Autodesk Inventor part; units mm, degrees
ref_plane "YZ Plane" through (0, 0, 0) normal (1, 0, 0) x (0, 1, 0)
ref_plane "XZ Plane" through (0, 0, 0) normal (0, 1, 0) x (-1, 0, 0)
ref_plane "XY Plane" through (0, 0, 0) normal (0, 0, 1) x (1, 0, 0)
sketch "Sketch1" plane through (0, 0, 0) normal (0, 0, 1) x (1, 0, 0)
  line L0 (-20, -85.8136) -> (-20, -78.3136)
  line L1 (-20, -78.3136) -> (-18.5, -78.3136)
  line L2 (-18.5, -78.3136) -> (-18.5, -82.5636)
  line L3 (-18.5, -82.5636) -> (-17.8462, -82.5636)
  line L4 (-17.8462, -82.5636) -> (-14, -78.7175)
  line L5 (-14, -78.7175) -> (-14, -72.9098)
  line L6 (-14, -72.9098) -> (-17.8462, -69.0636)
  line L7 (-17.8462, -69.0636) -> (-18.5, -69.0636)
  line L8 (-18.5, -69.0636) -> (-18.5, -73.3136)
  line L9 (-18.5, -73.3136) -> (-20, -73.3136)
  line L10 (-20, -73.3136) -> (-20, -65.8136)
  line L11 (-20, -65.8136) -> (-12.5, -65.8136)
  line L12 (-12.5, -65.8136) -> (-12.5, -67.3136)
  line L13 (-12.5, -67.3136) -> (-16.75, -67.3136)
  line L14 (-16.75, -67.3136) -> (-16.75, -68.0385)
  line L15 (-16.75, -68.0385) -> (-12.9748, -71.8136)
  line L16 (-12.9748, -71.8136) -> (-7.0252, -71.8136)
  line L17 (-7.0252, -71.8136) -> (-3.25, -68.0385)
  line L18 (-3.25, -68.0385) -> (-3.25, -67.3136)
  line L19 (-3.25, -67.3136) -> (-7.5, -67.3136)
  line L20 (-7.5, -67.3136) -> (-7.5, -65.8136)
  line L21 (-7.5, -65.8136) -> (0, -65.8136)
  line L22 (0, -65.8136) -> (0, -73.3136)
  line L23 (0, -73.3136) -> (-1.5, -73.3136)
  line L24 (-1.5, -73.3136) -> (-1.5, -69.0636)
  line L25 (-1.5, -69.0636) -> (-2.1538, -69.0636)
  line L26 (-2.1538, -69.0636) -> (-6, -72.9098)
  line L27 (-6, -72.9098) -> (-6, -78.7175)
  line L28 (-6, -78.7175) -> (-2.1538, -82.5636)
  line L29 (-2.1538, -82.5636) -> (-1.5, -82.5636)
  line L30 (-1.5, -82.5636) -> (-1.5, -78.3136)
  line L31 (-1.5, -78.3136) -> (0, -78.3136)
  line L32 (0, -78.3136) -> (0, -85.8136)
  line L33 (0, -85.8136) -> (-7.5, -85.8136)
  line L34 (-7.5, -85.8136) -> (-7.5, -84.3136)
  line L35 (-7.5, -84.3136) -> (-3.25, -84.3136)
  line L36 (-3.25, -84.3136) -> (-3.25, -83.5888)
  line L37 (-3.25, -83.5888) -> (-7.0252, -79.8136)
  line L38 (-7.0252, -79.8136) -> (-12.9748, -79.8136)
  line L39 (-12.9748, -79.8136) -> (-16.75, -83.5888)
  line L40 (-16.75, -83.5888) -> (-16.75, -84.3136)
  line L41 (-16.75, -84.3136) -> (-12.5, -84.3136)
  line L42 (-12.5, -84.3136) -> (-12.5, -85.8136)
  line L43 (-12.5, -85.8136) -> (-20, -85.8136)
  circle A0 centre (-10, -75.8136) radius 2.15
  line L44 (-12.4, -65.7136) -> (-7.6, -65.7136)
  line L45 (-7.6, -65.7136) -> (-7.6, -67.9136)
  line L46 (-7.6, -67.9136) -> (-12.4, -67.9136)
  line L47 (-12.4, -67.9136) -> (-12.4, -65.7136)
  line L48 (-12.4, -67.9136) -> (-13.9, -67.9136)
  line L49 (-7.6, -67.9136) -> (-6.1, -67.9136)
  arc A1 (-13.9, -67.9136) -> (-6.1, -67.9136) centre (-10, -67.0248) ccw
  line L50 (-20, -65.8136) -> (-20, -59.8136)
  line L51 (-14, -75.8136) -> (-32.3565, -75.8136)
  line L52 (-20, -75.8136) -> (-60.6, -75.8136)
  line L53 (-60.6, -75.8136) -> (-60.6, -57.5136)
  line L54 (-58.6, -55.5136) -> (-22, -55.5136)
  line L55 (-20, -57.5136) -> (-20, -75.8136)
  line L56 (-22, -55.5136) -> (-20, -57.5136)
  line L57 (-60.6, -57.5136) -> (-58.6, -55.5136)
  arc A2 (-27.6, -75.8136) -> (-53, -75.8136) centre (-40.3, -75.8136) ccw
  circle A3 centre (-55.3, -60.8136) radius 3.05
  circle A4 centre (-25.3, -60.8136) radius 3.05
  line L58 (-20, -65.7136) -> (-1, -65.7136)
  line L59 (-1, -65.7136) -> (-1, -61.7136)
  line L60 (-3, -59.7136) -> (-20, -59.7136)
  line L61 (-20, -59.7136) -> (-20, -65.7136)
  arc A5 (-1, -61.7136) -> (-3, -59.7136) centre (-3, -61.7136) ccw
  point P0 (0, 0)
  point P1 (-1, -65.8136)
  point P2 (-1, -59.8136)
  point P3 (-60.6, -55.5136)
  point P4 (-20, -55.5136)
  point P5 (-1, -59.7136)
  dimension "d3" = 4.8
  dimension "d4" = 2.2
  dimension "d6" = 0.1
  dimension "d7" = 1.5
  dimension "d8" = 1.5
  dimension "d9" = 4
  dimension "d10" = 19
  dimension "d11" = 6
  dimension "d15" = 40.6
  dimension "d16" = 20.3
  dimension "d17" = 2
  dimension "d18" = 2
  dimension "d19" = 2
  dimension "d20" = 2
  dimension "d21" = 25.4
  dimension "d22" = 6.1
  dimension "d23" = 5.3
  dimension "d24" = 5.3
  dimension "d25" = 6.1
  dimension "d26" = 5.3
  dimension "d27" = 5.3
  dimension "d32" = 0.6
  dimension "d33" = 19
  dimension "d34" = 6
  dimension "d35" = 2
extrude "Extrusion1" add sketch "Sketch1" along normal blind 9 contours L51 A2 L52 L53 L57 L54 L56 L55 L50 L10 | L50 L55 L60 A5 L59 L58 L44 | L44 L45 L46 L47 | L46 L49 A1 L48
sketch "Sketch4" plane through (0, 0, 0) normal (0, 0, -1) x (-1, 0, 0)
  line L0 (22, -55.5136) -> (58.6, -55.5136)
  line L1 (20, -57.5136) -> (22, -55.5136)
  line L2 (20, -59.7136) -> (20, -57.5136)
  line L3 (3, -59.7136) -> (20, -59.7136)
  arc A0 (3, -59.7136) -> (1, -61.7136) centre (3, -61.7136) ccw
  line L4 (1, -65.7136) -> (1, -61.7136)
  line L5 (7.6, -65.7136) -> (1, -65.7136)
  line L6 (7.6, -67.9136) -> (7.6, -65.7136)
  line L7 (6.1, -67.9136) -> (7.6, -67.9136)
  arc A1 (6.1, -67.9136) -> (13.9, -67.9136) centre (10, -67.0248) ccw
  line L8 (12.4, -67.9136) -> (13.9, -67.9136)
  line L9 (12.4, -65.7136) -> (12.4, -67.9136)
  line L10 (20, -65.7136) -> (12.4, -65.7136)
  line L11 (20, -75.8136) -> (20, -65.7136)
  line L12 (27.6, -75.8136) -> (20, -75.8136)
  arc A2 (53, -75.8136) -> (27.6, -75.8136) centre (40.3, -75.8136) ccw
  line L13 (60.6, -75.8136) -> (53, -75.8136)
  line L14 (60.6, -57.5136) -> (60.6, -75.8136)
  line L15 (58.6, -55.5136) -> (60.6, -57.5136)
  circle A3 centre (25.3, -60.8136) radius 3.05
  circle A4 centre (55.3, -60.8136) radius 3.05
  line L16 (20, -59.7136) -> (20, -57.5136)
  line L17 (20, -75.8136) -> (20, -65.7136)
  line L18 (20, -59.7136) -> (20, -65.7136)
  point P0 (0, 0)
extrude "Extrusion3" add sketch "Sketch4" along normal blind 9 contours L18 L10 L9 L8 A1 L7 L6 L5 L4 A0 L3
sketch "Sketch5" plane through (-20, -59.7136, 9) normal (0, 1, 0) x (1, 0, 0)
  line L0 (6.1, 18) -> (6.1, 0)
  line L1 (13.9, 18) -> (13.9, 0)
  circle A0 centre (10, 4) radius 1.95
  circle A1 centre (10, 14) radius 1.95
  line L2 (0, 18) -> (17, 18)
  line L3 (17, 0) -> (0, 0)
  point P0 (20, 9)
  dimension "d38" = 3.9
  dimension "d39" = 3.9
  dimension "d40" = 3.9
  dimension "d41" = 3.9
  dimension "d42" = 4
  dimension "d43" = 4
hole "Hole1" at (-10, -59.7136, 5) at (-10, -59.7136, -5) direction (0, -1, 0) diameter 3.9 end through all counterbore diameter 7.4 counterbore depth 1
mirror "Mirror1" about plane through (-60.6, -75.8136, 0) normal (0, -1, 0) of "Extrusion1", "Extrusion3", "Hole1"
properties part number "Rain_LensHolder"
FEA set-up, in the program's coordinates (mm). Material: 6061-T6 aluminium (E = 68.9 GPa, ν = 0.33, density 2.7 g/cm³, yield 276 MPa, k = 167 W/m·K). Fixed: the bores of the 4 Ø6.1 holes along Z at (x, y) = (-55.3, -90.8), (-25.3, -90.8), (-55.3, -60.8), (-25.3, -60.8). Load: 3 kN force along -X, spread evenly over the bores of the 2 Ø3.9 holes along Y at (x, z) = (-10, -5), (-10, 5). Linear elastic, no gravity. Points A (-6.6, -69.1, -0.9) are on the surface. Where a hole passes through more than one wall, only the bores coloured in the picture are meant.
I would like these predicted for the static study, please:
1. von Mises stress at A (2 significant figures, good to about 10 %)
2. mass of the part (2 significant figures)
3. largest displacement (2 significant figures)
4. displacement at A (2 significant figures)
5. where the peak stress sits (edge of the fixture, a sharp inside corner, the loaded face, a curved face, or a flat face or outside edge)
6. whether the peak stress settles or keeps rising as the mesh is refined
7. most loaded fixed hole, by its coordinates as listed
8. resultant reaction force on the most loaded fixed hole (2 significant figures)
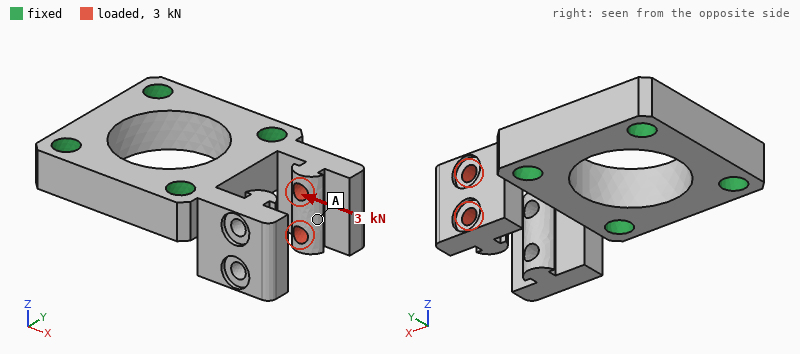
28 MPa
37 g
0.17 mm
0.13 mm
a sharp inside corner
keeps rising
(-25.3, -60.8)
2.8 kN
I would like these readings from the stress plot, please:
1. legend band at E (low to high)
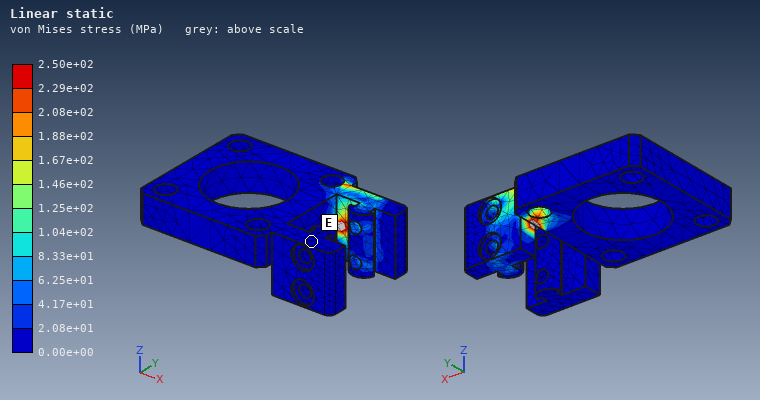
0.00e+00 to 2.08e+01 MPa
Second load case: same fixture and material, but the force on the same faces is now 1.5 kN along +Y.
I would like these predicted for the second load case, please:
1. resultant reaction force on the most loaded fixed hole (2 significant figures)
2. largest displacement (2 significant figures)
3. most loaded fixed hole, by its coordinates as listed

1.2 kN
0.19 mm
(-25.3, -60.8)
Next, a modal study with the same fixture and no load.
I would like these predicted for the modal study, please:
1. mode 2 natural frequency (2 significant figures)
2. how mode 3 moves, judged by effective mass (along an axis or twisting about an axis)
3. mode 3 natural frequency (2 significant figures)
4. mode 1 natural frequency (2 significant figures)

7300 Hz
along Z
9300 Hz
7300 Hz
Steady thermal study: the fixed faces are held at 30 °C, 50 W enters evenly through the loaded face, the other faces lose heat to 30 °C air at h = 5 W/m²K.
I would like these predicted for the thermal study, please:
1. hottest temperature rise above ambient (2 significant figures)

65 K
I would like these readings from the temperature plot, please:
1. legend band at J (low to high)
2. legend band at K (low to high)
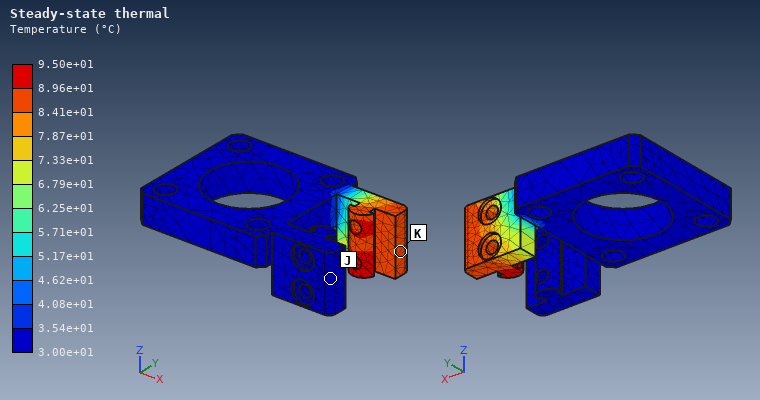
3.00e+01 to 3.54e+01 °C
8.41e+01 to 8.96e+01 °C
